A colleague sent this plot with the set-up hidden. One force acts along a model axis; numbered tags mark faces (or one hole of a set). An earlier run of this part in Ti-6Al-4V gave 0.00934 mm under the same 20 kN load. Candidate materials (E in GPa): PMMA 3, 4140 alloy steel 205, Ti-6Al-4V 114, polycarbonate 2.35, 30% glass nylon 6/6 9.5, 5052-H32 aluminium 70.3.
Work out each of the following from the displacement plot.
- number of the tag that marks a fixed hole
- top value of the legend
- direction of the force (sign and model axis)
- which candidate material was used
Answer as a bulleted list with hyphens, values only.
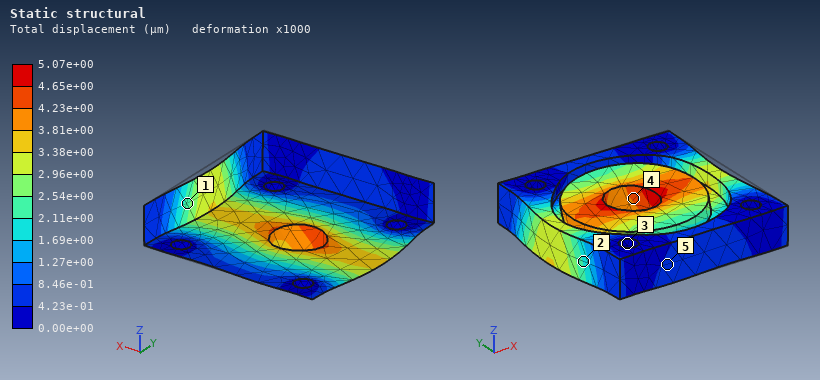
- 3
- 5.07e+00 µm
- -X
- 4140 alloy steel
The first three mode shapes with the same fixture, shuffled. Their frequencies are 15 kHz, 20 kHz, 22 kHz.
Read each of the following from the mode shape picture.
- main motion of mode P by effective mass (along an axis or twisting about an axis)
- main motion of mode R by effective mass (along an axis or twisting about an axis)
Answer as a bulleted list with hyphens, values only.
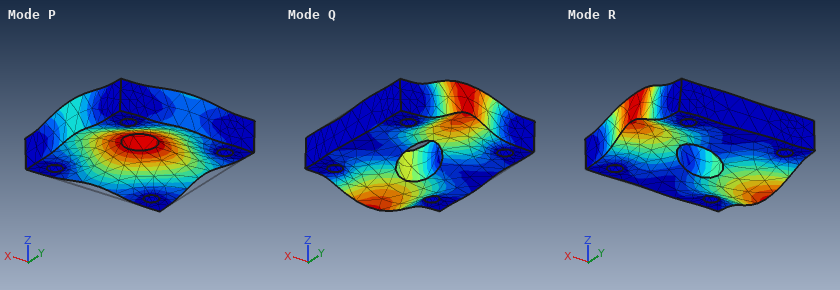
- along Z
- twisting about Y
